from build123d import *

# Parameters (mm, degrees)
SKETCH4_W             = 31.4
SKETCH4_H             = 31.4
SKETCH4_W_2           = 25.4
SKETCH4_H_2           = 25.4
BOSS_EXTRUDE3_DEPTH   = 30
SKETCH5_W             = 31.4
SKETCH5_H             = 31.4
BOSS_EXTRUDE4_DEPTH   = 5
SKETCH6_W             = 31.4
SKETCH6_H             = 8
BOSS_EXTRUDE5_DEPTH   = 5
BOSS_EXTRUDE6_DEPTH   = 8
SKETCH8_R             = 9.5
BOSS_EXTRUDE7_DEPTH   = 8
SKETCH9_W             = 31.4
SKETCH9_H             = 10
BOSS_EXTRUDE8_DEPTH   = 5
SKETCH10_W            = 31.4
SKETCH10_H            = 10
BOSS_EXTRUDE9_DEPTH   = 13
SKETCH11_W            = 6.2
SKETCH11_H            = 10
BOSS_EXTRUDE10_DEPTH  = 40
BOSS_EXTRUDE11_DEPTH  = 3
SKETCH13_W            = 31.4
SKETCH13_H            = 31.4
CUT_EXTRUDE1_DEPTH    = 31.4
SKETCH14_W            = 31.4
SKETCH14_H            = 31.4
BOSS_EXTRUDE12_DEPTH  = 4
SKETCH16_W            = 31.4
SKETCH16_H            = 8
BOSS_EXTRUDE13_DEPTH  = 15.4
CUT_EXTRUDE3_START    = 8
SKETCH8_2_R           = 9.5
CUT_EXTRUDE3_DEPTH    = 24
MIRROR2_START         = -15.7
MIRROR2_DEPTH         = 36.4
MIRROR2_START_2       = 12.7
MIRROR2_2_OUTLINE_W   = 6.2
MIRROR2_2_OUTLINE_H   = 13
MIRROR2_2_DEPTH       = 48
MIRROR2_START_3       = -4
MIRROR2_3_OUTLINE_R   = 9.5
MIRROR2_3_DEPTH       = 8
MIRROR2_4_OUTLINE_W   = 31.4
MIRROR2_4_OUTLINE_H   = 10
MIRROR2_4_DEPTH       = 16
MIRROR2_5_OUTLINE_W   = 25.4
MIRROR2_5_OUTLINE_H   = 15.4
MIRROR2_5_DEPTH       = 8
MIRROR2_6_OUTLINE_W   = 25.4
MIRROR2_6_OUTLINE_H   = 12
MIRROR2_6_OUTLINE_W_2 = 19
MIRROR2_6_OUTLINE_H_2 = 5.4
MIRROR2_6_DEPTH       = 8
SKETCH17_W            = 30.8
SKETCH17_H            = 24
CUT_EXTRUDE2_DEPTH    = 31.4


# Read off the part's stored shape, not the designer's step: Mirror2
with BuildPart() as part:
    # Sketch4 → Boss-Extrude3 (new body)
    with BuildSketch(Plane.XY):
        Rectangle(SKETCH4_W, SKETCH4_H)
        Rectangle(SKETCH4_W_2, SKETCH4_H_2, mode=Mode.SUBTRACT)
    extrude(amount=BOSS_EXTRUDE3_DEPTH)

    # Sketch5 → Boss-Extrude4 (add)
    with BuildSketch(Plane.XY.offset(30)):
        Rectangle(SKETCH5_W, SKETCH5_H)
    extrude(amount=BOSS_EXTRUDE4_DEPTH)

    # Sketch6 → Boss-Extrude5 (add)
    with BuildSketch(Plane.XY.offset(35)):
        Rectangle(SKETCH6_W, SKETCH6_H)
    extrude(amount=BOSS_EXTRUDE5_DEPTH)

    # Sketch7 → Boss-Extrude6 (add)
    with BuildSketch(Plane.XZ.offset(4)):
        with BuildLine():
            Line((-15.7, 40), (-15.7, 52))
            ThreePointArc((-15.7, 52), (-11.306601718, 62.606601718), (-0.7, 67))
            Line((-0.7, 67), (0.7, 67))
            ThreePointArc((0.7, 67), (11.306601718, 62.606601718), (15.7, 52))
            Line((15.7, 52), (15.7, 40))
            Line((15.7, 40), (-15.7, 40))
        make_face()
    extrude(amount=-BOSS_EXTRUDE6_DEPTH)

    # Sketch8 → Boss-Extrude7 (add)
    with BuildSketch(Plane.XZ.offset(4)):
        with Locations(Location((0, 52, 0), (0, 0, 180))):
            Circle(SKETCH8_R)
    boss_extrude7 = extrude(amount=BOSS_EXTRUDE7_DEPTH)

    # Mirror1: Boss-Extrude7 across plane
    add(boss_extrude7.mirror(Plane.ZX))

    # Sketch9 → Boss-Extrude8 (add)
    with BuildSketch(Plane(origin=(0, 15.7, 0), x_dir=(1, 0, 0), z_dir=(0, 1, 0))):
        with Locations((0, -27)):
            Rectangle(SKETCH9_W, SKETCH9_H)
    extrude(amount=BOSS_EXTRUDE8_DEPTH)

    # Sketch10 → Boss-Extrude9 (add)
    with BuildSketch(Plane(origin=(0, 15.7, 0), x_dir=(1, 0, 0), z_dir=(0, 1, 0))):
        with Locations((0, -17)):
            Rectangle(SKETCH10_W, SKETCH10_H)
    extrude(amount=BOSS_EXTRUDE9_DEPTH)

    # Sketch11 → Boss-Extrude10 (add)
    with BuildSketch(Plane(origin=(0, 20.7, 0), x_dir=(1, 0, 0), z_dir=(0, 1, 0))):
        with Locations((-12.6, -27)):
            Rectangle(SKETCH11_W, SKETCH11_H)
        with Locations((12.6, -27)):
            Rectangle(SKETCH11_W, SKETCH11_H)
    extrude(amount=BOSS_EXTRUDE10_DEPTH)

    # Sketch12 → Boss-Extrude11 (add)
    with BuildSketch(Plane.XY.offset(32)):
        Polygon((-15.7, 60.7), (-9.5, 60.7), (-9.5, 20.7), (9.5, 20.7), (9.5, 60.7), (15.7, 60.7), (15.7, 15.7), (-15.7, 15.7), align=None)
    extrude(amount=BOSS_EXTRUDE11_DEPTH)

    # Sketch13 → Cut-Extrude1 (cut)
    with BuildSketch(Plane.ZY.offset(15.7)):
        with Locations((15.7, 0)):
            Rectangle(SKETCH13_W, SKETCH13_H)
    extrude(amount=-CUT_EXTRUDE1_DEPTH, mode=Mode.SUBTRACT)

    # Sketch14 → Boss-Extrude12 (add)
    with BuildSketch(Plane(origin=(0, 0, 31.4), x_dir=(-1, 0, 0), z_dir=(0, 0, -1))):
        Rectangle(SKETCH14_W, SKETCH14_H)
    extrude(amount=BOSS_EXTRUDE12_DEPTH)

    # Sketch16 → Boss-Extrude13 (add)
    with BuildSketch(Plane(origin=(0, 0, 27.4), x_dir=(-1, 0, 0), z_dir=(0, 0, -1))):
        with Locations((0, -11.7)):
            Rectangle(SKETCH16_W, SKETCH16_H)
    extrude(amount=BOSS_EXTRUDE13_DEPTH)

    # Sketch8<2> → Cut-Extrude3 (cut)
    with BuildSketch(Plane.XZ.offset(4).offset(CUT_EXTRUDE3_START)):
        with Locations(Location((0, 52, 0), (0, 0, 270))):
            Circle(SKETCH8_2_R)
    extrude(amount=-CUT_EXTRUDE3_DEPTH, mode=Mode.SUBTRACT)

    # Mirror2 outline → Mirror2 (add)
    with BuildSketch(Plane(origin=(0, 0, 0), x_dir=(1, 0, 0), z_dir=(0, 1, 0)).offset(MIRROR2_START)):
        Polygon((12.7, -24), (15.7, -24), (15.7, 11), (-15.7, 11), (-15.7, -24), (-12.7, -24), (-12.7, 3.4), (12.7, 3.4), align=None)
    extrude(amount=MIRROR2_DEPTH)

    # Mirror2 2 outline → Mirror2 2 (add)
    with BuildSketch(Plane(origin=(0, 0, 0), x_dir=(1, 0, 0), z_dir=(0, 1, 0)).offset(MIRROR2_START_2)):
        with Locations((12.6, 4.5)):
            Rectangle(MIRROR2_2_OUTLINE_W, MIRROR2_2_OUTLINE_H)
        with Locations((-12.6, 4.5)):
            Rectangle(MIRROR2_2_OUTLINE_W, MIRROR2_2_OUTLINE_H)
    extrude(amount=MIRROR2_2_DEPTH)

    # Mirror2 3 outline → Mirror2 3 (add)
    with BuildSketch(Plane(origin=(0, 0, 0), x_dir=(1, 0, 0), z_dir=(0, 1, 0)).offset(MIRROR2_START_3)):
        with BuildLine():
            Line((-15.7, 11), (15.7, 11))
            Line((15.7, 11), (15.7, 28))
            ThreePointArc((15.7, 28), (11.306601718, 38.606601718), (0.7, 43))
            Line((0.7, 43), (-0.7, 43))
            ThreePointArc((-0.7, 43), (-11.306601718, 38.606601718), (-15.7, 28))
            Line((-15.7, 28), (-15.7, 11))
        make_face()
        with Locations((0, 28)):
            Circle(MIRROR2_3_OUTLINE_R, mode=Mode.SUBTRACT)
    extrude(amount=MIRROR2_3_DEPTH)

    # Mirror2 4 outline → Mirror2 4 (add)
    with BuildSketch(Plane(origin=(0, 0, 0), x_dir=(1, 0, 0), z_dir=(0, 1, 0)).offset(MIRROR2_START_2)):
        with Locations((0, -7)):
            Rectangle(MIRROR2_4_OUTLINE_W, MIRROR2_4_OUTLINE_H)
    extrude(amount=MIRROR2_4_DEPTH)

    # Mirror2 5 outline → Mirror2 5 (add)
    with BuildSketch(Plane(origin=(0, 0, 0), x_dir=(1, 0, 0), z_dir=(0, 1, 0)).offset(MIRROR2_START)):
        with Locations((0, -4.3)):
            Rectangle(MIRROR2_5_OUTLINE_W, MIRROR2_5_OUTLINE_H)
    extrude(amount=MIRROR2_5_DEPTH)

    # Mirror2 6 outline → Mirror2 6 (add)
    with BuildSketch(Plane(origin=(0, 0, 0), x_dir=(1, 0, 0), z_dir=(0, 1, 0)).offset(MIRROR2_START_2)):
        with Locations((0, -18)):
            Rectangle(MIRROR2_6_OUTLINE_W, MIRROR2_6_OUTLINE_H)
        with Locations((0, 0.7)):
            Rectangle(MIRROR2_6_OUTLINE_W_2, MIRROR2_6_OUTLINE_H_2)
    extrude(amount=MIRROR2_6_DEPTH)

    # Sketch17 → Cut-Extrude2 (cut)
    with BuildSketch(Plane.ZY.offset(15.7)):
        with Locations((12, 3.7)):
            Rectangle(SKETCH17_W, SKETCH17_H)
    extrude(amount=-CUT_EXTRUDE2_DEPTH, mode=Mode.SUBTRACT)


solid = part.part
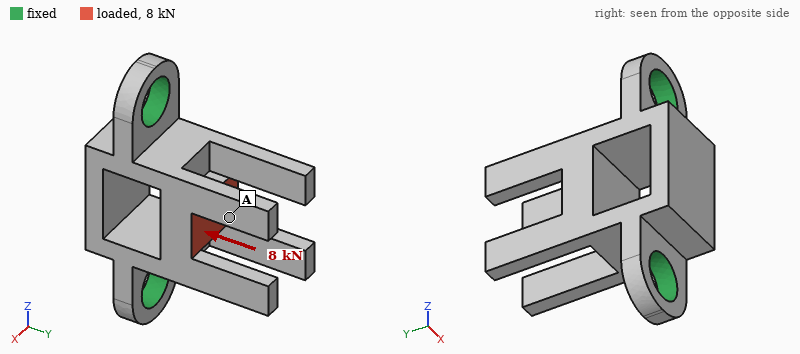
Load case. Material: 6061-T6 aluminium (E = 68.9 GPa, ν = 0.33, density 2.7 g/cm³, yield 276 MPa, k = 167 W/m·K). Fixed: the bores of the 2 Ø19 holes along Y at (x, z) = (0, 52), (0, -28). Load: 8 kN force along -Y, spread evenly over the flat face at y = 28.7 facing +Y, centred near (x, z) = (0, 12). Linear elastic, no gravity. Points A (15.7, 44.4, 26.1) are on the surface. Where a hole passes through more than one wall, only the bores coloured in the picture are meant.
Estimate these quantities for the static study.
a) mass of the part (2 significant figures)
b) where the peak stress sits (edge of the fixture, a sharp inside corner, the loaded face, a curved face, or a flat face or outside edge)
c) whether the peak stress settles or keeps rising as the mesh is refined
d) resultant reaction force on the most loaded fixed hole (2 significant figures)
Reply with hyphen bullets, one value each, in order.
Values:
- 150 g
- edge of the fixture
- keeps rising
- 4.1 kN
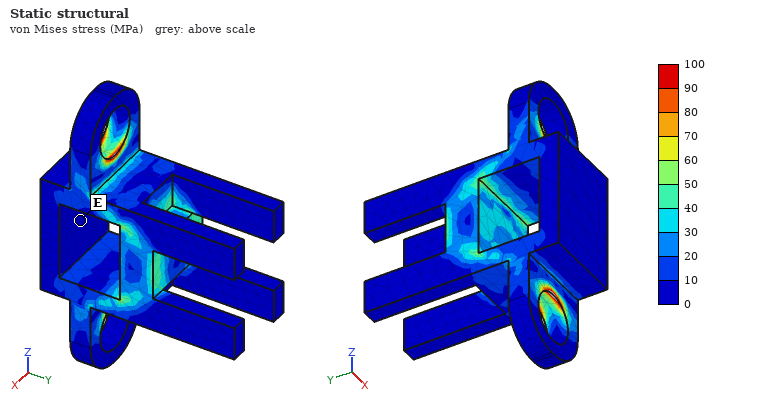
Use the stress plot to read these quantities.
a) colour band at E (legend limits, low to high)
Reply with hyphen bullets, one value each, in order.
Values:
- 0 to 10 MPa
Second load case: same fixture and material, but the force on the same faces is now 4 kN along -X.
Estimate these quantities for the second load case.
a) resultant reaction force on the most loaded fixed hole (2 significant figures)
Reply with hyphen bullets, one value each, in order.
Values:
- 2.0 kN
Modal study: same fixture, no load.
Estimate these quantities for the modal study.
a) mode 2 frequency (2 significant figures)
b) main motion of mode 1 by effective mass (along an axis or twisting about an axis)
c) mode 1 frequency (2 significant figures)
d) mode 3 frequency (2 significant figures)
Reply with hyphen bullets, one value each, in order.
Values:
- 3100 Hz
- along X
- 2300 Hz
- 3200 Hz
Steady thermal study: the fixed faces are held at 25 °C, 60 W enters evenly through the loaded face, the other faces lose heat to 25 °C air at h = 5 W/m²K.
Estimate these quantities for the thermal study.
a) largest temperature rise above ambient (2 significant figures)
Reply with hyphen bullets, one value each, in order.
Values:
- 32 K
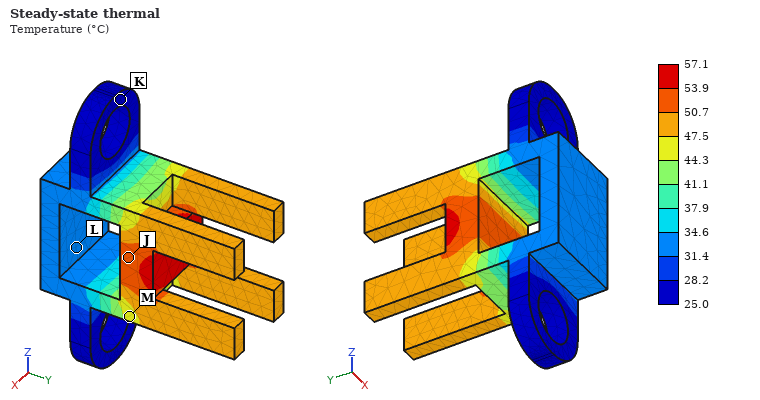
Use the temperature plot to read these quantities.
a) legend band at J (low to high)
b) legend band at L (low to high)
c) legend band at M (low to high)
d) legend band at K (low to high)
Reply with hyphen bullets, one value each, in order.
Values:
- 50.7 to 53.9 °C
- 31.4 to 34.6 °C
- 44.3 to 47.5 °C
- 25.0 to 28.2 °C
